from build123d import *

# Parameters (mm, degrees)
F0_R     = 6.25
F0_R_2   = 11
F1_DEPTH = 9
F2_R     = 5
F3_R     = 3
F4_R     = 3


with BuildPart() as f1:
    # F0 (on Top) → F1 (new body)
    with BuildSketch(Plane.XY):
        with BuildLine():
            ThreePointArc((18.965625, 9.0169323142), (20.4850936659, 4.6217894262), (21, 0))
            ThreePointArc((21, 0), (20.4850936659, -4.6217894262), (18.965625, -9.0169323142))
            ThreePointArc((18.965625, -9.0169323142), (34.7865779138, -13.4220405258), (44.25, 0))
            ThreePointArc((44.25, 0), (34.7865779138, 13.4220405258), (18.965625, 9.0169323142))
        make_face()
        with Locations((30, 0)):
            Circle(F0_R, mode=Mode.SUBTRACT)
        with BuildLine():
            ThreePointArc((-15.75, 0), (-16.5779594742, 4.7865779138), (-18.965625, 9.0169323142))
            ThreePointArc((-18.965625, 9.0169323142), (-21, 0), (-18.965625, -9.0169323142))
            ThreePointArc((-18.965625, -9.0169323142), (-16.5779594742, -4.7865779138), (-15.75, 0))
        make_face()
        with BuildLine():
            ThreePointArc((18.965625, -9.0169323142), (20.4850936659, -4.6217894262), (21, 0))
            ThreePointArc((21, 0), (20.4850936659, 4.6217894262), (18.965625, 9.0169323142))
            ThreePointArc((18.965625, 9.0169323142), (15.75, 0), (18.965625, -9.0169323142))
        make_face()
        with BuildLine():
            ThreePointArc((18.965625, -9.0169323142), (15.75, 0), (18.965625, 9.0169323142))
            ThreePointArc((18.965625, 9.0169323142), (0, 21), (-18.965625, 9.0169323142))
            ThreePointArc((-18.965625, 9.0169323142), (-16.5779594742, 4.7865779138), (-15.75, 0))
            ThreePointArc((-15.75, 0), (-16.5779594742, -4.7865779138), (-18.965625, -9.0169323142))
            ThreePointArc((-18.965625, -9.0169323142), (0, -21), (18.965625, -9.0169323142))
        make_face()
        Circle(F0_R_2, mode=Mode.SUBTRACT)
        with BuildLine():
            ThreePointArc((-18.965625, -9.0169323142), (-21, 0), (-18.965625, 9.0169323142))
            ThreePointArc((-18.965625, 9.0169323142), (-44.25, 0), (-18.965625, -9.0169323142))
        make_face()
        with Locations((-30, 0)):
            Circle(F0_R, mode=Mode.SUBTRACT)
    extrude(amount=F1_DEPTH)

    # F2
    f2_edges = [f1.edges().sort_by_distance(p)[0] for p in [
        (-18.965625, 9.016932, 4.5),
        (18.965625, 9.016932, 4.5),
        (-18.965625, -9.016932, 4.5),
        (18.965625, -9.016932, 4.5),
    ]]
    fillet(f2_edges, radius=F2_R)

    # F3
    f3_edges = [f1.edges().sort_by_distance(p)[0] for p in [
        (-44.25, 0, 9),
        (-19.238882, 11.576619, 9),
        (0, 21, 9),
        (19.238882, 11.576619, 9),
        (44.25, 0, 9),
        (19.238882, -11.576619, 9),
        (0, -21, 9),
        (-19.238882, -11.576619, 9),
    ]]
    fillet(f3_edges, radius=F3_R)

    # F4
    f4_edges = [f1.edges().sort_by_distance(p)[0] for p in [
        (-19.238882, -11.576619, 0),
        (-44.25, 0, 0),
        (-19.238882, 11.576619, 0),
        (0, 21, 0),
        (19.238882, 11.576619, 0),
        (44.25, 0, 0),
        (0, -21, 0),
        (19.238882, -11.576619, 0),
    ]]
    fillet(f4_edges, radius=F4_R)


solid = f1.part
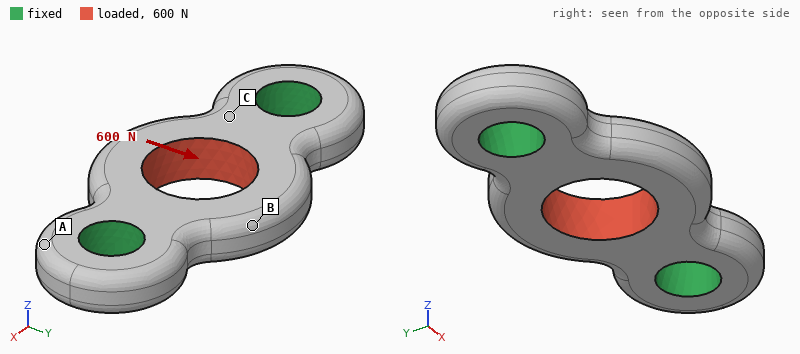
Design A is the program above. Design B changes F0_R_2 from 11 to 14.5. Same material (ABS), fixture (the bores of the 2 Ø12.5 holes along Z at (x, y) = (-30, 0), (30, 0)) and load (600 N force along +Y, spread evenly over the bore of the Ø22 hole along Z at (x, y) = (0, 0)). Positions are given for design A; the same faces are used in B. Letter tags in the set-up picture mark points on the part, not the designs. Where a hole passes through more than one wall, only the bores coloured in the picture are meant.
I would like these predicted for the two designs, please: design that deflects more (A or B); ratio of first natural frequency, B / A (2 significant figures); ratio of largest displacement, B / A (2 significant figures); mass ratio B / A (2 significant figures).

B
1.0
1.1
0.85
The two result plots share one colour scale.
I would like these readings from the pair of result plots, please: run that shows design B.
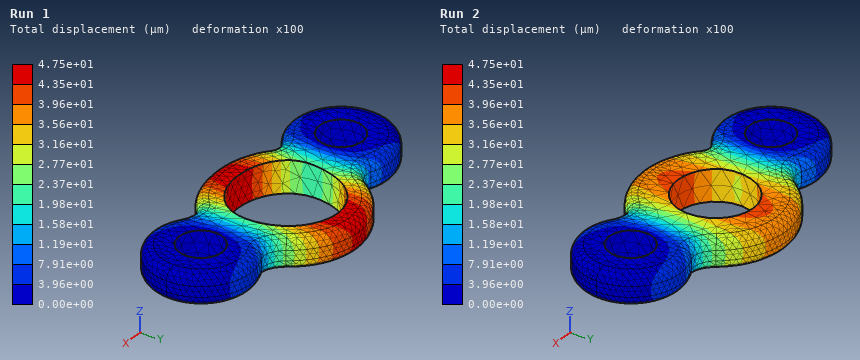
Run 1
